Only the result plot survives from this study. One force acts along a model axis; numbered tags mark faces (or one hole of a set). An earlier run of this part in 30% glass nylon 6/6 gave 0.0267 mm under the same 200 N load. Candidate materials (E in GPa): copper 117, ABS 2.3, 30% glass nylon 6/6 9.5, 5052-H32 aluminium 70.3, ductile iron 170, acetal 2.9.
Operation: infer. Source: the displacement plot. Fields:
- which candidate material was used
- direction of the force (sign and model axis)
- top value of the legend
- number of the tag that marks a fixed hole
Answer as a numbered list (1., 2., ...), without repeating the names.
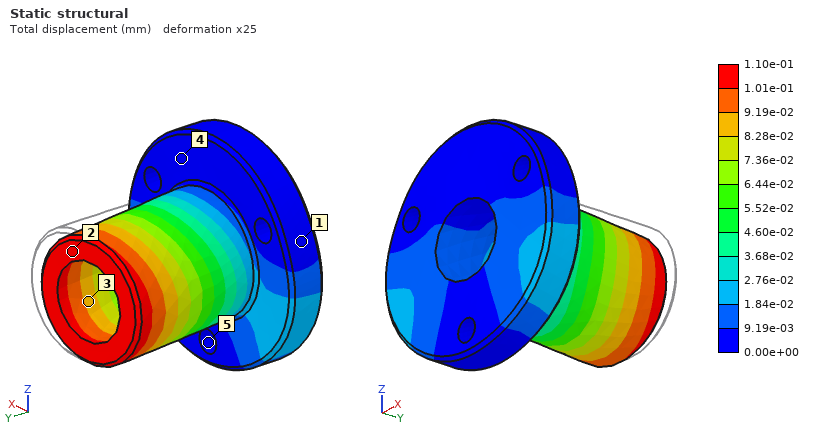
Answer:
1. ABS
2. -X
3. 1.10e-01 mm
4. 5
